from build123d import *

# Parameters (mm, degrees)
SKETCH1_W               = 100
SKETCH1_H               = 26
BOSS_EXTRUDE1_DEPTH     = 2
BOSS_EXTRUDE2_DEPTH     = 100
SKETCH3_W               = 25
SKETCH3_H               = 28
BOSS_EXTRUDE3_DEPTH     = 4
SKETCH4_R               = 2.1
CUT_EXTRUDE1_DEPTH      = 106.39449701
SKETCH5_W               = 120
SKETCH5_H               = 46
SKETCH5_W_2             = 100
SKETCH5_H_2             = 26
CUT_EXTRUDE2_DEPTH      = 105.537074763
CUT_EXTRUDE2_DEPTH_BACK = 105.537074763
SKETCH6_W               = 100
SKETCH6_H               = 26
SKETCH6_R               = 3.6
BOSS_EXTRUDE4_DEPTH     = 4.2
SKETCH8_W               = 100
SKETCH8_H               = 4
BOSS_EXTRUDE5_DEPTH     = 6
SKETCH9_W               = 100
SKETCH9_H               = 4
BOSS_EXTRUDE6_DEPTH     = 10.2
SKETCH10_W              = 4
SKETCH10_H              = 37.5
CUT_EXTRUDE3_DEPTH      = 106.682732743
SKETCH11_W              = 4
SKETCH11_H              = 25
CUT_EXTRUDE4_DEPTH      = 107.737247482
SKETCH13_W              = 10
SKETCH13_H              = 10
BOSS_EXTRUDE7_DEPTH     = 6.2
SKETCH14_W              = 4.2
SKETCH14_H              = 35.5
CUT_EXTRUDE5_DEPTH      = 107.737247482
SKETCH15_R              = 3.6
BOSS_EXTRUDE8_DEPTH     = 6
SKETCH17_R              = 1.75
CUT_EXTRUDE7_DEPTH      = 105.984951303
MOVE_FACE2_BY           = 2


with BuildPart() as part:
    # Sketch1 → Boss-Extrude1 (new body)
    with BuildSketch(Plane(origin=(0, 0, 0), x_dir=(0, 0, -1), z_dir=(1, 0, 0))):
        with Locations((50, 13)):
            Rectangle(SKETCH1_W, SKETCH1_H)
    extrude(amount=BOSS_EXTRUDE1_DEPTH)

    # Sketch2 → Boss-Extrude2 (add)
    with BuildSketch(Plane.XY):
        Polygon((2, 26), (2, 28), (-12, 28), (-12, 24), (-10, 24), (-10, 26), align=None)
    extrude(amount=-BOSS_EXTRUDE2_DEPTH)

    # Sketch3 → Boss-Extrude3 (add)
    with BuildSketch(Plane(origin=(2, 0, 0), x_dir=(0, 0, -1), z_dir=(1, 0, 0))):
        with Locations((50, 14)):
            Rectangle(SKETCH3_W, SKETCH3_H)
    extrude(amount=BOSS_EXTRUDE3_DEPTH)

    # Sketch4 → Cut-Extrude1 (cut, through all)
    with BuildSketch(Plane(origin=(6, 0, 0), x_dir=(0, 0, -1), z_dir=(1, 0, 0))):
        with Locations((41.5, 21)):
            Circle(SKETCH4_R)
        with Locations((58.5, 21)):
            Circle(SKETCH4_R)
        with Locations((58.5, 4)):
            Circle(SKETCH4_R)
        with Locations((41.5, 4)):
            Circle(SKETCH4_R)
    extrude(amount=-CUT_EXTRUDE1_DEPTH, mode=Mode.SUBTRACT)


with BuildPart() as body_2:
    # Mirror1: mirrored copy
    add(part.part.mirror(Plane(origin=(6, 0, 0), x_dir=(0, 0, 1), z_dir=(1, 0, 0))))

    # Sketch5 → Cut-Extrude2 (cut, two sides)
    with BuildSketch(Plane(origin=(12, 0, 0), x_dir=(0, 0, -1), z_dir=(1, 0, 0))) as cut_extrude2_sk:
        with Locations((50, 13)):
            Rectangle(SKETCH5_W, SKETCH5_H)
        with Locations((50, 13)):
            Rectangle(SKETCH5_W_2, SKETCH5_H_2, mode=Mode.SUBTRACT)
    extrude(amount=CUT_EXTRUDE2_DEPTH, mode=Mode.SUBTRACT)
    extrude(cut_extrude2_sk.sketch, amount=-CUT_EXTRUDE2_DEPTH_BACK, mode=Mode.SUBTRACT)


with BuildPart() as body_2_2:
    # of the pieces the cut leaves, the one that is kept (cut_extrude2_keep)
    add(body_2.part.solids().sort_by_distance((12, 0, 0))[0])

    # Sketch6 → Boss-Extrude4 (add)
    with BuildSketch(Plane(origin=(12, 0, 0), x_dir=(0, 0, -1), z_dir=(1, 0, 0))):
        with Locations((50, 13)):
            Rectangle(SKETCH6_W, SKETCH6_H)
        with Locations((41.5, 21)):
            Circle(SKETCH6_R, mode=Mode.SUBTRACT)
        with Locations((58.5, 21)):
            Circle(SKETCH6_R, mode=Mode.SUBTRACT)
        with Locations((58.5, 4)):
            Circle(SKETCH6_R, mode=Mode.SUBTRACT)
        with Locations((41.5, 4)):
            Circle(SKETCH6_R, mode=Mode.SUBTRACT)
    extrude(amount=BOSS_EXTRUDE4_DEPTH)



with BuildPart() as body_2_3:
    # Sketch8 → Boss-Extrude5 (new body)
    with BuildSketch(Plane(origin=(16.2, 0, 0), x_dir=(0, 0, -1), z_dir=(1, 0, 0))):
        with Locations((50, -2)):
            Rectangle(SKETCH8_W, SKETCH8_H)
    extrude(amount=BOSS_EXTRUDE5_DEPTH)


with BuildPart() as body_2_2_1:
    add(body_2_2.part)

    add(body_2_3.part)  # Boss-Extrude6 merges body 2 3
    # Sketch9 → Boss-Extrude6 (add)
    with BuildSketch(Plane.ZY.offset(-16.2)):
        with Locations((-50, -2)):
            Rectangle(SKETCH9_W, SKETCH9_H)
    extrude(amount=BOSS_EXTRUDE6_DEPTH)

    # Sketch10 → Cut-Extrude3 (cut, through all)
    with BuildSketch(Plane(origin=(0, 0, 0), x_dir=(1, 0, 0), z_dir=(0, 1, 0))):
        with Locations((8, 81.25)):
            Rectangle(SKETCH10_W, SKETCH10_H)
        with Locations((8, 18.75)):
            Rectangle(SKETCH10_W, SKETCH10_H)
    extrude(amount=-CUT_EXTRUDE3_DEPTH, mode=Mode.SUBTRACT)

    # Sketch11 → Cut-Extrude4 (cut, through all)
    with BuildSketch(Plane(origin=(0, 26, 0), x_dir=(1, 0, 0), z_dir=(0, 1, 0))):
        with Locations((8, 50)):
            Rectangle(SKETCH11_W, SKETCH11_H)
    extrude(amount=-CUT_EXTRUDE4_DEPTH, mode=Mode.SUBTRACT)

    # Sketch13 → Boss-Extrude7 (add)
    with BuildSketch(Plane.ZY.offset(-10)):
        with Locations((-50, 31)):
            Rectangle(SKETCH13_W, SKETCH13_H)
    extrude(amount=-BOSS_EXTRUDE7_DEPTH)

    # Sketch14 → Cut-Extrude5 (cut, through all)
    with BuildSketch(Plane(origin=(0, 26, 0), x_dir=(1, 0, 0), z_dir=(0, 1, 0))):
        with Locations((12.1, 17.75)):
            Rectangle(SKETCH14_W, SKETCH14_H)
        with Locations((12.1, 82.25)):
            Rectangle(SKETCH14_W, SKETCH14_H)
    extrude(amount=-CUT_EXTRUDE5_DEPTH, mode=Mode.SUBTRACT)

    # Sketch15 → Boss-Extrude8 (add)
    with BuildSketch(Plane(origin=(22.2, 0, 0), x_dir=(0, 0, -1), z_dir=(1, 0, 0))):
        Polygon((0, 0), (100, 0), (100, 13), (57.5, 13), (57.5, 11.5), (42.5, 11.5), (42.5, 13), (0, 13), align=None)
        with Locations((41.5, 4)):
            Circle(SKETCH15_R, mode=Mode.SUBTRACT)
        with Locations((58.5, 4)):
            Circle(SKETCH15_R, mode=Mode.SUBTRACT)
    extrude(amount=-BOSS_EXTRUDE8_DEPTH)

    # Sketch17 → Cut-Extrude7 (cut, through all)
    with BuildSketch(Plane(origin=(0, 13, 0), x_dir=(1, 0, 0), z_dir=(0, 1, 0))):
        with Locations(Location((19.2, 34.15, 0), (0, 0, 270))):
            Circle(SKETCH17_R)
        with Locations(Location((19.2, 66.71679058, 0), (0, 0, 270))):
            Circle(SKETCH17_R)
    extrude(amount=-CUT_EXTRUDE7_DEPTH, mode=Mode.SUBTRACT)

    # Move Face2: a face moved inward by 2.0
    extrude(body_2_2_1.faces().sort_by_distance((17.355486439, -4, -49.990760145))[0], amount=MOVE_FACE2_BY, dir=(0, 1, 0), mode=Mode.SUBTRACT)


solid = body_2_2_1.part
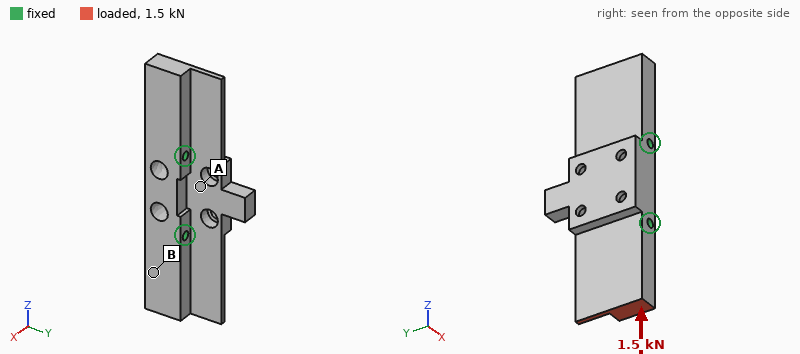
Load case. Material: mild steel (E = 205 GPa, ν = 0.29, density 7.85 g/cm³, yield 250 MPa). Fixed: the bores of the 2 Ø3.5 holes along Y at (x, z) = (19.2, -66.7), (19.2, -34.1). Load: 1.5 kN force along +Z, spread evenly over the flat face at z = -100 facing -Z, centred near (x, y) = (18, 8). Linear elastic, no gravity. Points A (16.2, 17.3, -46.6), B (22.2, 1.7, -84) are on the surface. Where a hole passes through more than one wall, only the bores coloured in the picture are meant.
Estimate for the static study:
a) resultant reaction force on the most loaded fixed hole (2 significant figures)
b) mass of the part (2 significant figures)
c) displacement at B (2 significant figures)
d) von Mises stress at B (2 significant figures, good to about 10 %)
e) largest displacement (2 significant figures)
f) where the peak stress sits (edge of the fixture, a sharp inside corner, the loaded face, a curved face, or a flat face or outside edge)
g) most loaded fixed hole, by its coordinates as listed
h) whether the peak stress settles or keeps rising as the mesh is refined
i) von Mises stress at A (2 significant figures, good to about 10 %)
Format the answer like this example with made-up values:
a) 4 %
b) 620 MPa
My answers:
a) 1.4 kN
b) 130 g
c) 0.95 µm
d) 9.8 MPa
e) 2.9 µm
f) edge of the fixture
g) (19.2, -66.7)
h) keeps rising
i) 2.1 MPa
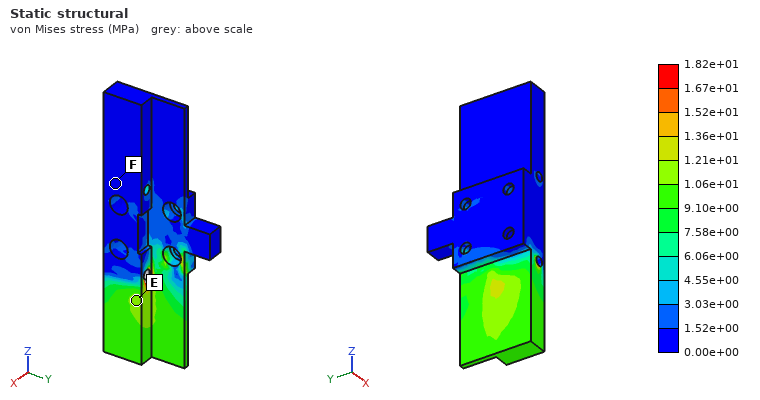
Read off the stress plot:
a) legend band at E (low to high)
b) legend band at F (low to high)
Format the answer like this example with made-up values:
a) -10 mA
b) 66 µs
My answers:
a) 1.06e+01 to 1.21e+01 MPa
b) 0.00e+00 to 1.52e+00 MPa
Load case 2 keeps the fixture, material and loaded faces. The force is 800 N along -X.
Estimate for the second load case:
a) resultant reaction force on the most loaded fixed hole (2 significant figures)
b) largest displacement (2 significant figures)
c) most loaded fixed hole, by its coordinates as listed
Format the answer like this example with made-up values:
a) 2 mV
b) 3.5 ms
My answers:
a) 1.2 kN
b) 0.11 mm
c) (19.2, -66.7)
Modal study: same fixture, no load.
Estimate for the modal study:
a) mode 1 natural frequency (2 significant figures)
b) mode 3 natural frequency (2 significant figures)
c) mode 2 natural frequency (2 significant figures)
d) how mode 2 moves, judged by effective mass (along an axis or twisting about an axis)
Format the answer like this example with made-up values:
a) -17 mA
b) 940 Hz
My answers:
a) 4800 Hz
b) 8200 Hz
c) 5000 Hz
d) along X
